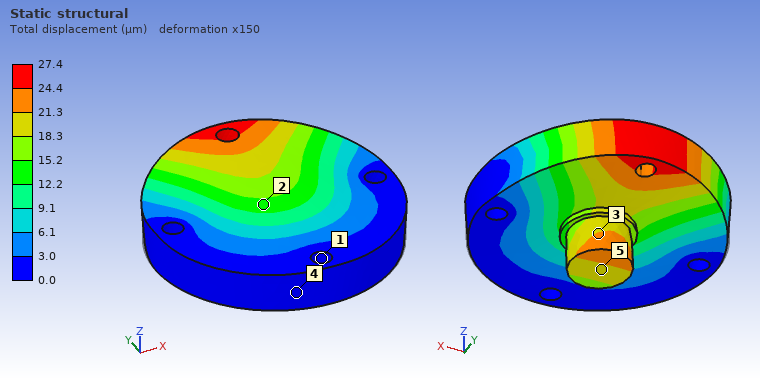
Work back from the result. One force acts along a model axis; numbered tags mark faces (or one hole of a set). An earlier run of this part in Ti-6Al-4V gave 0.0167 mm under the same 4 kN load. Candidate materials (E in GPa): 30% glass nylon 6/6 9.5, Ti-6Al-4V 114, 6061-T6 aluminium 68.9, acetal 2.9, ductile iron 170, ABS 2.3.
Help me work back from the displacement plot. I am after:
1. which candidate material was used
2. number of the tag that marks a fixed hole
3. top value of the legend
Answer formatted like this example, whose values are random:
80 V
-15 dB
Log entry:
6061-T6 aluminium
1
27.4 µm
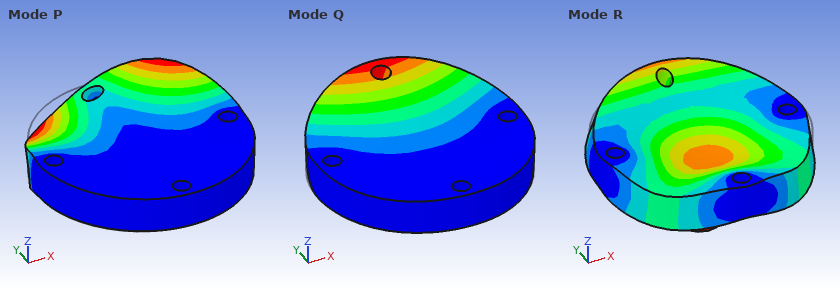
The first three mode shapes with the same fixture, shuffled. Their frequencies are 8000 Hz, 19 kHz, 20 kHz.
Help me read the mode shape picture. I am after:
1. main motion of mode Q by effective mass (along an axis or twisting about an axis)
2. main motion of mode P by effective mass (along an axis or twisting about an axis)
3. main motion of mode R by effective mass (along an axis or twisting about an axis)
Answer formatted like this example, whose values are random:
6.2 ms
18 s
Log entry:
along Z
twisting about Y
along Z
